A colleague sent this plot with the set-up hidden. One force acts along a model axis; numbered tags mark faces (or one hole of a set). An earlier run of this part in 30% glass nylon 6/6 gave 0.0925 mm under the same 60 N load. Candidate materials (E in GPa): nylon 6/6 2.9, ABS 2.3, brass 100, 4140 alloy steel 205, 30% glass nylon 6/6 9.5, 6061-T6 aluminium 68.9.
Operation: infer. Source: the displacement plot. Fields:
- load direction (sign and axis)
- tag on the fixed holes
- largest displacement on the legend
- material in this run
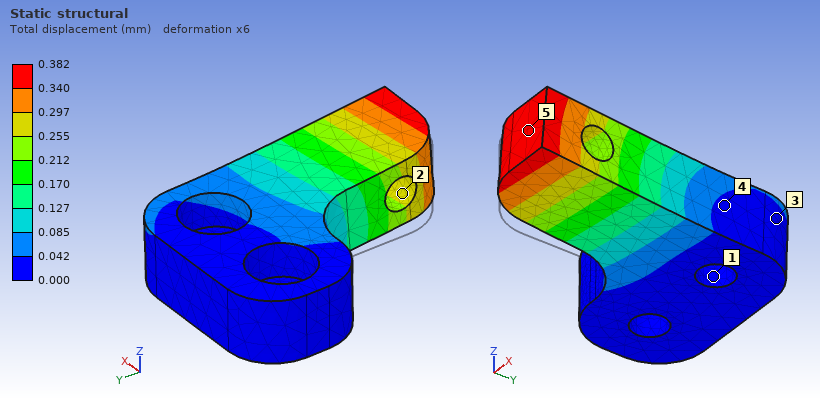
+Z
1
0.382 mm
ABS
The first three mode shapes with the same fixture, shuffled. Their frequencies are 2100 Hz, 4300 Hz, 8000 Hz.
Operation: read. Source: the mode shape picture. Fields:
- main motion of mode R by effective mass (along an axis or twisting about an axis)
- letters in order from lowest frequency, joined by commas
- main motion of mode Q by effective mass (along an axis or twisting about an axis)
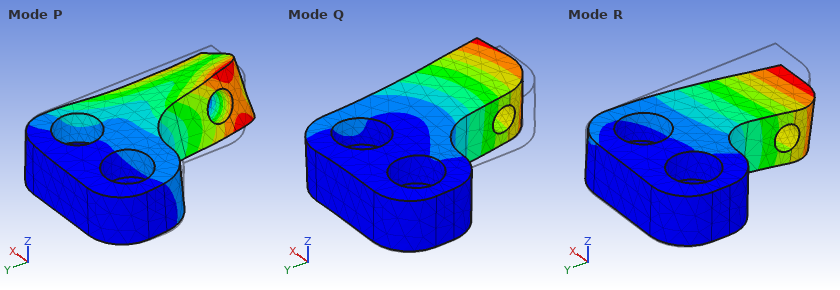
along Z
R, Q, P
along X
